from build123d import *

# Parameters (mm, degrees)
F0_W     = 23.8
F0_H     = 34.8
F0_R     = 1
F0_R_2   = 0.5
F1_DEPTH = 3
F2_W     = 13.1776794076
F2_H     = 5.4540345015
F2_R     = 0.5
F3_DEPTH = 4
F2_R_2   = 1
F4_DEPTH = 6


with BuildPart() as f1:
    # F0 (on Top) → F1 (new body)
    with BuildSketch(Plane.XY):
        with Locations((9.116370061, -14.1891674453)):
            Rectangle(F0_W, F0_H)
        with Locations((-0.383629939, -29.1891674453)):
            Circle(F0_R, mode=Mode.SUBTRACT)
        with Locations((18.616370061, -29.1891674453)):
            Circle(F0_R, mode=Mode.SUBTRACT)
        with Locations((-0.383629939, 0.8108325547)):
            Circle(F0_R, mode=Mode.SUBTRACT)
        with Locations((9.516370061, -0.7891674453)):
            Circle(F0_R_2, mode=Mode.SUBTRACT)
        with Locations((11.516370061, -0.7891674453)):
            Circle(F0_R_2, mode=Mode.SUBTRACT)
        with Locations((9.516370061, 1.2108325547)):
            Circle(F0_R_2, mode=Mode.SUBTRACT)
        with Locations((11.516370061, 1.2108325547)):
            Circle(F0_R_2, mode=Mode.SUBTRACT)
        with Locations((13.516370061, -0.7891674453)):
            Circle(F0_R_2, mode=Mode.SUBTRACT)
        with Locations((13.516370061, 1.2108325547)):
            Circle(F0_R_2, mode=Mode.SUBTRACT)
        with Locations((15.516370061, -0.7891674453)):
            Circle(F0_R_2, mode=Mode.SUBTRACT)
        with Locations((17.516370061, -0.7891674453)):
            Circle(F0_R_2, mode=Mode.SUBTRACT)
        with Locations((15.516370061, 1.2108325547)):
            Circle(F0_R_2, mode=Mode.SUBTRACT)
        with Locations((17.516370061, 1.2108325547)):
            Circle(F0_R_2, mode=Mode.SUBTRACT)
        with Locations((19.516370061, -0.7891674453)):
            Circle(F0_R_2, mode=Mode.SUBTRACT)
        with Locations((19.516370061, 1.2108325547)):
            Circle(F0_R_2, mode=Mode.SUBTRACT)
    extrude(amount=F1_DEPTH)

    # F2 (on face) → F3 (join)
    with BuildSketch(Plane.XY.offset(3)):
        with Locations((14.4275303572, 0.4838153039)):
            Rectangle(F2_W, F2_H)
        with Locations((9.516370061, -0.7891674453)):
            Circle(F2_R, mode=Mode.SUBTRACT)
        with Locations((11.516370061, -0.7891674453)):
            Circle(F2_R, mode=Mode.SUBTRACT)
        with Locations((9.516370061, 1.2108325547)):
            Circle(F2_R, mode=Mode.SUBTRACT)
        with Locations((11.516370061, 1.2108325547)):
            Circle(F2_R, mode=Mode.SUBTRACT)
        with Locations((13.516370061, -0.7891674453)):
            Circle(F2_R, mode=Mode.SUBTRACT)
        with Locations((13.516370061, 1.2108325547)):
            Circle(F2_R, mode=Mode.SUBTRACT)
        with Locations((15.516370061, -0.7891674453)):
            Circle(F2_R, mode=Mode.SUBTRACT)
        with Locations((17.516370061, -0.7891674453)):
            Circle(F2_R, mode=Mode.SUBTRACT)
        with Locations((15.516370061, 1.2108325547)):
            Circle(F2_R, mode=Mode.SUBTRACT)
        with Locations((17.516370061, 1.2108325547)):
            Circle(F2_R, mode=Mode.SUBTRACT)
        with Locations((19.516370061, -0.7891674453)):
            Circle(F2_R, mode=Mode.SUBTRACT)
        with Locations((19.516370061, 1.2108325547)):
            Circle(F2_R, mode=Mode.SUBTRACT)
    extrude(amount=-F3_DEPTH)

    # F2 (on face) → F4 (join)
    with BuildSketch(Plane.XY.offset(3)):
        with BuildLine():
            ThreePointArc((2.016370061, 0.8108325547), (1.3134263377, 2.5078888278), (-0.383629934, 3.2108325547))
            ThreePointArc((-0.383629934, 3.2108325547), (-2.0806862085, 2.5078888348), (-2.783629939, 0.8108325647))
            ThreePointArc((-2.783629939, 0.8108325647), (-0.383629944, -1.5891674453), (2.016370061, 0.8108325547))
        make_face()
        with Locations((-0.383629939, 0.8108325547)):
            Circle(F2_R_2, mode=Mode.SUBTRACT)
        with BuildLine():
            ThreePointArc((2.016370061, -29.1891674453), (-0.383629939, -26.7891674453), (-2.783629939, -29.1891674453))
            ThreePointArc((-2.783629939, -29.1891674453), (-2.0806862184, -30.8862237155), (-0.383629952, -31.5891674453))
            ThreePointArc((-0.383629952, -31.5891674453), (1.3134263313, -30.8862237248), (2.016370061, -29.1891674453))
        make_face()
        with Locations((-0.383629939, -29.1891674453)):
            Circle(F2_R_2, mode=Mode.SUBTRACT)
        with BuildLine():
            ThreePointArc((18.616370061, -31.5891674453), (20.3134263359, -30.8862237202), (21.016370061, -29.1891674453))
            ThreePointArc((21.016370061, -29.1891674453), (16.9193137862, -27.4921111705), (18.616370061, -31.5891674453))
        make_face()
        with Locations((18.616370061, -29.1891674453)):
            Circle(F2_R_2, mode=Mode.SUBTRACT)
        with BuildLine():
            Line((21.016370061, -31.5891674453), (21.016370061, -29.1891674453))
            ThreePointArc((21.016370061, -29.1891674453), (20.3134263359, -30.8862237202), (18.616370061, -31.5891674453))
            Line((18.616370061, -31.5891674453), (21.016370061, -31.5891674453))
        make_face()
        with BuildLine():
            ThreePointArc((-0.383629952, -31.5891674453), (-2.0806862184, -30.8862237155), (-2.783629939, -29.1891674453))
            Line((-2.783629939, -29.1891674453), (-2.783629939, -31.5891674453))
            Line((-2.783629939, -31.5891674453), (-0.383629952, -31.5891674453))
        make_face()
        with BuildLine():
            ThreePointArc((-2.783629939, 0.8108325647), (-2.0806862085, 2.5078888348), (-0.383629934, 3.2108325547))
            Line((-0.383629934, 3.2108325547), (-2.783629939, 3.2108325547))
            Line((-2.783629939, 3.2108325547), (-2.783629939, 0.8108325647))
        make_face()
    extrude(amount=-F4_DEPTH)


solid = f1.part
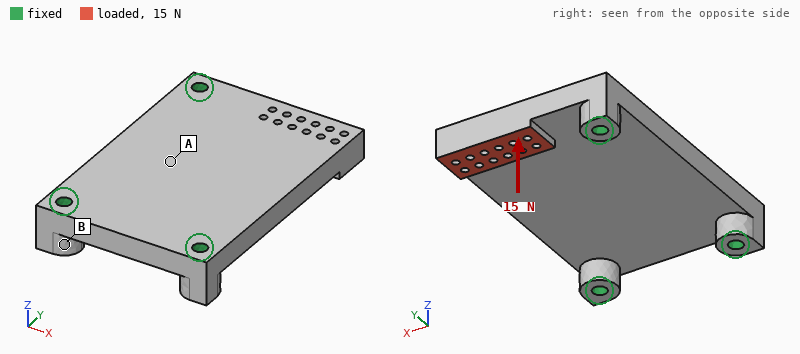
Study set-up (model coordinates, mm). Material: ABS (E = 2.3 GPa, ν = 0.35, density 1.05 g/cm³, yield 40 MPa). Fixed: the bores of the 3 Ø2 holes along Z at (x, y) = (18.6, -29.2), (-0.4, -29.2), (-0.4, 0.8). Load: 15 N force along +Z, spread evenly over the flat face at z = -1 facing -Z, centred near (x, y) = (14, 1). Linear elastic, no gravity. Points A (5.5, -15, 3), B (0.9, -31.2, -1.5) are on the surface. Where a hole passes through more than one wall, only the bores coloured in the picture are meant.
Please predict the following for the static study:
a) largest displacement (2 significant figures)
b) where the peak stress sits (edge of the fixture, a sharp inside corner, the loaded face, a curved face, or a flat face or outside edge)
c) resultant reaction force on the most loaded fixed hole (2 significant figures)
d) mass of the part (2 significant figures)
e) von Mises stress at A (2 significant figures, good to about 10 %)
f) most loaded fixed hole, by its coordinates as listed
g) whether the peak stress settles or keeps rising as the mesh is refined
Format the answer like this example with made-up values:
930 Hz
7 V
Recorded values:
0.27 mm
edge of the fixture
14 N
2.8 g
1.7 MPa
(-0.4, 0.8)
keeps rising
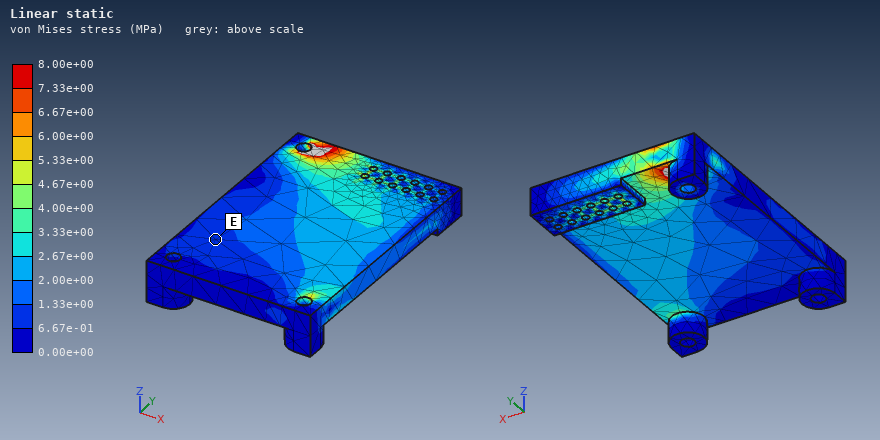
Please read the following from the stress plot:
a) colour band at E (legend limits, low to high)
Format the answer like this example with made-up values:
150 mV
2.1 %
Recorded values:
6.67e-01 to 1.33e+00 MPa
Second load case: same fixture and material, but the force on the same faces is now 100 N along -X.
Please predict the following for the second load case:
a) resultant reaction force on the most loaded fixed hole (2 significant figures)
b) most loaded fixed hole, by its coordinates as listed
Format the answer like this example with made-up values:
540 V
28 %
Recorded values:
90 N
(-0.4, 0.8)
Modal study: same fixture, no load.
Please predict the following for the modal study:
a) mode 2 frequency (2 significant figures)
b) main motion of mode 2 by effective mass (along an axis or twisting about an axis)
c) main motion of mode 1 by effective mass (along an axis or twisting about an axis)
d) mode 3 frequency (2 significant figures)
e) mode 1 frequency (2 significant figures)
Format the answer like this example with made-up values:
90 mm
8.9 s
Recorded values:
4500 Hz
along Z
along Z
6500 Hz
2000 Hz
